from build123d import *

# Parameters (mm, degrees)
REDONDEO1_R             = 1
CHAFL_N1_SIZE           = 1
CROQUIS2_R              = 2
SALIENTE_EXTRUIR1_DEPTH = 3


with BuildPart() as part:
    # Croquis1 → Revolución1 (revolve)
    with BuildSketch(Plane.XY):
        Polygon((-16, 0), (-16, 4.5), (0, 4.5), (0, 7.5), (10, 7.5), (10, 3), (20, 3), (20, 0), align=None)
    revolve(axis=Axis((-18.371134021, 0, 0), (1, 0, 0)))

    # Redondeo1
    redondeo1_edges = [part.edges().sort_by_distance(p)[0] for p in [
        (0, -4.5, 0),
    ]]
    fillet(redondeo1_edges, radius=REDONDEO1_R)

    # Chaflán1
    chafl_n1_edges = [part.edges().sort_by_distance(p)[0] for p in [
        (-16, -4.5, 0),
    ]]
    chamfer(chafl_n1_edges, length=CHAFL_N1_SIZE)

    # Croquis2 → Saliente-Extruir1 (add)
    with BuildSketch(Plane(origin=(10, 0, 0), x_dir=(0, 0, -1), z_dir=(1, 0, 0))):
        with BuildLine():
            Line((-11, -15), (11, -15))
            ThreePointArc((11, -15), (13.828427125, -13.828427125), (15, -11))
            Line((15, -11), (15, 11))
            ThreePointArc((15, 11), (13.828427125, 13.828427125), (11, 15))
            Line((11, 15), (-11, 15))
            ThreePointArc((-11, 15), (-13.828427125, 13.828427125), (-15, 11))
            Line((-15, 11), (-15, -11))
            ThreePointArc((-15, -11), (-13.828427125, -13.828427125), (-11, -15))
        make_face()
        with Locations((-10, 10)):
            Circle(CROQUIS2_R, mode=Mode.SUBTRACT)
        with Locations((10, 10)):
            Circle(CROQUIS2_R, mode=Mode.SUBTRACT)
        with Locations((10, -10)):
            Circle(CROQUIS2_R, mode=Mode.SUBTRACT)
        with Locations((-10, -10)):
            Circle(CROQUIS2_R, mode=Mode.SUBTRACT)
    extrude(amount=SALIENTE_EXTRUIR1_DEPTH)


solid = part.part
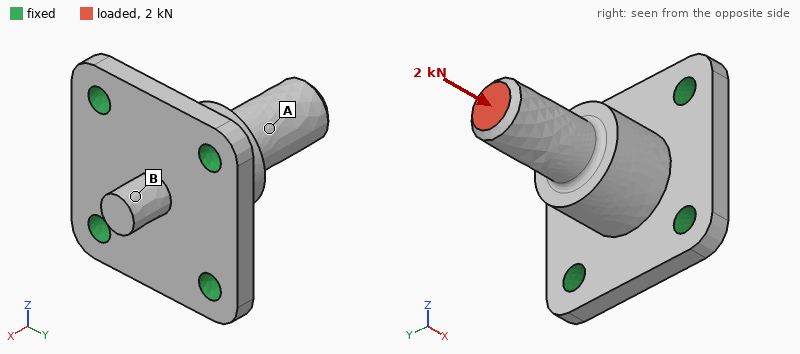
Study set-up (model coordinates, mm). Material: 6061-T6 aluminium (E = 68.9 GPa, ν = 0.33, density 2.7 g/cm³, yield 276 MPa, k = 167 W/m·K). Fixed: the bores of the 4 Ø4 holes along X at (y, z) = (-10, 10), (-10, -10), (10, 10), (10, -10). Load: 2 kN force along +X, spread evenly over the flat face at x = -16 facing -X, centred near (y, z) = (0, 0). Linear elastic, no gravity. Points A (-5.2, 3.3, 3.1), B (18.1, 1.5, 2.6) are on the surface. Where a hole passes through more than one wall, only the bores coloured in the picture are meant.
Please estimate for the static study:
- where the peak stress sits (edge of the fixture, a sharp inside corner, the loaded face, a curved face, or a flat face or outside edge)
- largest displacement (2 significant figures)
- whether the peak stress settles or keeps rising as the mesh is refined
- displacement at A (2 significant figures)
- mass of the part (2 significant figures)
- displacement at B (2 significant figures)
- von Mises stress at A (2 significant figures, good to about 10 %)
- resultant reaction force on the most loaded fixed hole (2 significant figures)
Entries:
edge of the fixture
23 µm
keeps rising
17 µm
15 g
13 µm
31 MPa
520 N
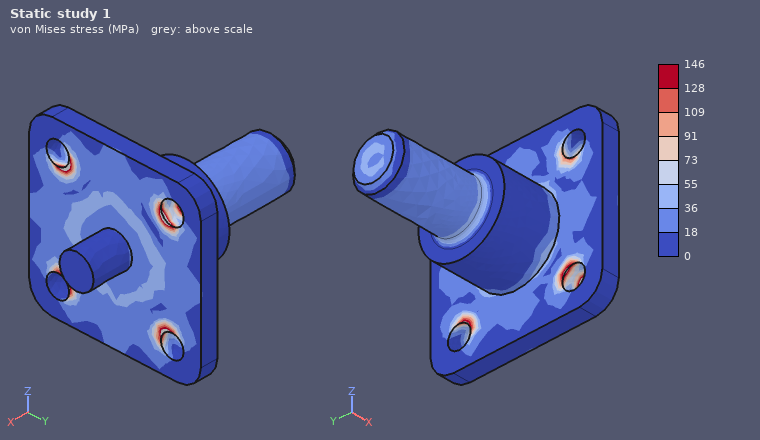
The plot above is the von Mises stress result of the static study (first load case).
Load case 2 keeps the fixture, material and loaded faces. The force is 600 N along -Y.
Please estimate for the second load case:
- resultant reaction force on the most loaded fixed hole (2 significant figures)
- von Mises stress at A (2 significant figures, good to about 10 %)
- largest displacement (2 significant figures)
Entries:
530 N
67 MPa
0.12 mm
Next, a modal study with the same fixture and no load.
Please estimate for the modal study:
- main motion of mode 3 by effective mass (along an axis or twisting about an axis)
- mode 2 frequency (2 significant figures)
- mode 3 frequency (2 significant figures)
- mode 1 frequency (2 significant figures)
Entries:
along X
10 kHz
19 kHz
10 kHz
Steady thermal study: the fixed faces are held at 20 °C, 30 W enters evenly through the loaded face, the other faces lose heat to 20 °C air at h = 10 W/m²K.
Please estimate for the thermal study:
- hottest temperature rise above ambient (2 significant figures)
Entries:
70 K
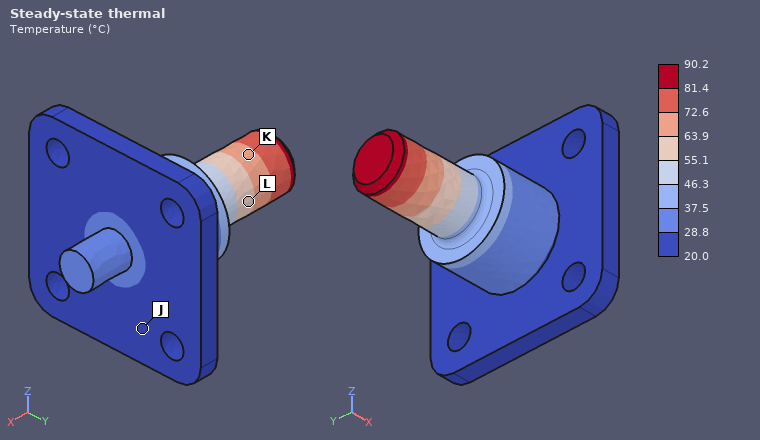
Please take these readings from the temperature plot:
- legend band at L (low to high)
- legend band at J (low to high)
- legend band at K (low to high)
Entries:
55.1 to 63.9 °C
20.0 to 28.8 °C
63.9 to 72.6 °C
